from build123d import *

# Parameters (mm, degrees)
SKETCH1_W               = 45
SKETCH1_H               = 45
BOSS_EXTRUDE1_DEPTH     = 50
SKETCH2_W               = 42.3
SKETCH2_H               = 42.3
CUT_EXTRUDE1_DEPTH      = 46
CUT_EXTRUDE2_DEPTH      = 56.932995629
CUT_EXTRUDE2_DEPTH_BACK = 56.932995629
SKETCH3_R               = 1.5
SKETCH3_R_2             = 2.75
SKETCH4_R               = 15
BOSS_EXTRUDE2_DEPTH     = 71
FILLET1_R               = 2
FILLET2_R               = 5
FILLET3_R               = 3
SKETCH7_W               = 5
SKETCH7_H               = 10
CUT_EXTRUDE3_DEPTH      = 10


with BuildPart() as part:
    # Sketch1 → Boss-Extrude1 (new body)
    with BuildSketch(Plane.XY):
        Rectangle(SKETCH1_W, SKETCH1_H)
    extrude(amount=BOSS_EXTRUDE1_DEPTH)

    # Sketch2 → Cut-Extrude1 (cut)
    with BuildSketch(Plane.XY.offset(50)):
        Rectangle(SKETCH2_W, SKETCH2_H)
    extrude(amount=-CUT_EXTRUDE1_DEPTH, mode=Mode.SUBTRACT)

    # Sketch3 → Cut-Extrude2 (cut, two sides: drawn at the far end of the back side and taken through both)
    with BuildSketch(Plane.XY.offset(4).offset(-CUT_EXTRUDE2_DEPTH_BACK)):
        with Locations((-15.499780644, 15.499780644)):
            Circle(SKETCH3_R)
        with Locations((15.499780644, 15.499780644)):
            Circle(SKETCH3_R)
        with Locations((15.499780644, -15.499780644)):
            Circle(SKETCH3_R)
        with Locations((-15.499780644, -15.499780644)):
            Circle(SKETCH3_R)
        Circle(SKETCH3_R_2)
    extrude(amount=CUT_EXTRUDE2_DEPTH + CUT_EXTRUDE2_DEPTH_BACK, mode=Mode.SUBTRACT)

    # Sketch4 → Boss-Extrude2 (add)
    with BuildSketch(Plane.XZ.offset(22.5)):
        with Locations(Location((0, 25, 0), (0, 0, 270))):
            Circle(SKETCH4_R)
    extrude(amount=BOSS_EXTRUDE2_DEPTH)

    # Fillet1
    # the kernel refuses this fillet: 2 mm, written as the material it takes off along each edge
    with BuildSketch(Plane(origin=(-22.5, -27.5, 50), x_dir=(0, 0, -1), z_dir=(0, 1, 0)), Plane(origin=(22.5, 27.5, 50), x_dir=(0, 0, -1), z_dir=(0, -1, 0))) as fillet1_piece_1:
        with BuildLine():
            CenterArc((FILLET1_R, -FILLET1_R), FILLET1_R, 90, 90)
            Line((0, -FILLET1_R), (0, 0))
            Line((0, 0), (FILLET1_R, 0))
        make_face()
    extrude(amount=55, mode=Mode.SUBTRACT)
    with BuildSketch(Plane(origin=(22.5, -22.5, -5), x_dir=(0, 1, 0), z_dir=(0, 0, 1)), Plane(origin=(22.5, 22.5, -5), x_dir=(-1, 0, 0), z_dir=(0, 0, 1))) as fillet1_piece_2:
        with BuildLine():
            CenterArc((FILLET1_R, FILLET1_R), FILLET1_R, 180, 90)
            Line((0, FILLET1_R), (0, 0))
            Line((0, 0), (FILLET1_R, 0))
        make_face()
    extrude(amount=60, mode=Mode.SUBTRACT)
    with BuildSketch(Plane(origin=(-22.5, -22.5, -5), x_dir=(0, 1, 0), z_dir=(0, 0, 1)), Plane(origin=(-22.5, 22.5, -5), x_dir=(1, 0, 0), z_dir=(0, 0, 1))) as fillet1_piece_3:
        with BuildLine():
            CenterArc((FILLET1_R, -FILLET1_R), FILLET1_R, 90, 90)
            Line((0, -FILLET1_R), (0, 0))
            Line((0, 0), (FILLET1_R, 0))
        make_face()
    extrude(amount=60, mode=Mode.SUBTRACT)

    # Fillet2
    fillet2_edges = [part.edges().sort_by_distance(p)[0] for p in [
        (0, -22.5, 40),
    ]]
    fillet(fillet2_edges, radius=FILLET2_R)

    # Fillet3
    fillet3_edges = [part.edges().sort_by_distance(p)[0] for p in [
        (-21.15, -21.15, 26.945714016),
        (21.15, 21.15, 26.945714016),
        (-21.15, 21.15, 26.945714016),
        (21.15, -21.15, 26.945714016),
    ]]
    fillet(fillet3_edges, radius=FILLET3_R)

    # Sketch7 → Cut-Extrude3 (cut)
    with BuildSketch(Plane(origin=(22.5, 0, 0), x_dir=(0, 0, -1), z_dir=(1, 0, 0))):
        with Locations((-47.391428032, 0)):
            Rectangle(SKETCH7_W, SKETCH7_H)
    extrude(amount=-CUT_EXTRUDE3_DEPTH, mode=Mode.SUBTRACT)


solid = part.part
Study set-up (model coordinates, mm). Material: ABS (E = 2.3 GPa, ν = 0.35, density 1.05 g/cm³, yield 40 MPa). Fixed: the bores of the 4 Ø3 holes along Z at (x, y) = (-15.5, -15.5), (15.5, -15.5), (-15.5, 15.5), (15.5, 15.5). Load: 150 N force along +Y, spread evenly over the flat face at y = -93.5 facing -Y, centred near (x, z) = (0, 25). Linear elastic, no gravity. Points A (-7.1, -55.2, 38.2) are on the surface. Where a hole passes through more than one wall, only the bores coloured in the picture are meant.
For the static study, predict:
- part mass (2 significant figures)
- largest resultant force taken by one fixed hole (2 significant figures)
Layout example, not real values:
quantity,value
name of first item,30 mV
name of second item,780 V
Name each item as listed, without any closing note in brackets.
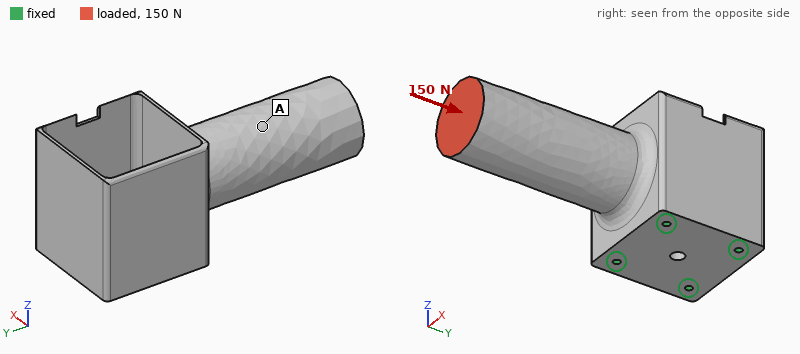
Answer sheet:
quantity,value
part mass,73 g
largest resultant force taken by one fixed hole,64 N
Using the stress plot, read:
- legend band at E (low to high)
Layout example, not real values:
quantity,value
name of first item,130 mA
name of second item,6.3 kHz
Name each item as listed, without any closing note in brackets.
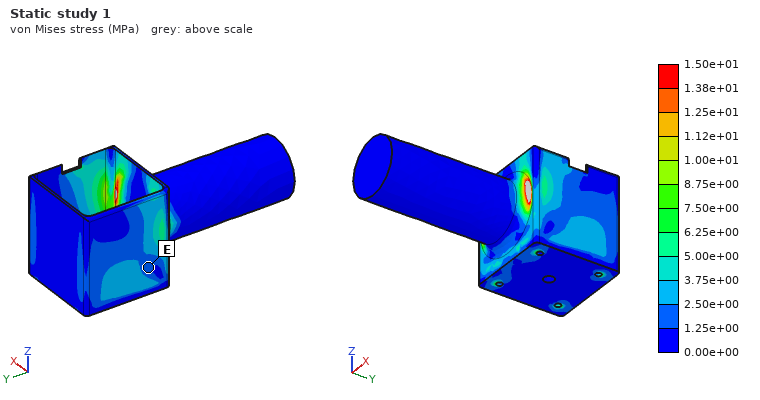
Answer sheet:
quantity,value
legend band at E,1.25e+00 to 2.50e+00 MPa
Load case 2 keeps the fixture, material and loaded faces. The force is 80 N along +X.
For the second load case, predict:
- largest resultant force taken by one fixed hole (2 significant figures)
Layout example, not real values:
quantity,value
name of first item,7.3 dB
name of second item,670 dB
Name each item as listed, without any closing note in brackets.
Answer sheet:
quantity,value
largest resultant force taken by one fixed hole,120 N
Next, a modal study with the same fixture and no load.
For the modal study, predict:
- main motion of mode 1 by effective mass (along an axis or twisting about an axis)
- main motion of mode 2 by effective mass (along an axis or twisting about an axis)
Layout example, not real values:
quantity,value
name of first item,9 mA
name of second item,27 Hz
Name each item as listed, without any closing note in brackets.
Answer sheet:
quantity,value
main motion of mode 1 by effective mass,along Z
main motion of mode 2 by effective mass,along X
